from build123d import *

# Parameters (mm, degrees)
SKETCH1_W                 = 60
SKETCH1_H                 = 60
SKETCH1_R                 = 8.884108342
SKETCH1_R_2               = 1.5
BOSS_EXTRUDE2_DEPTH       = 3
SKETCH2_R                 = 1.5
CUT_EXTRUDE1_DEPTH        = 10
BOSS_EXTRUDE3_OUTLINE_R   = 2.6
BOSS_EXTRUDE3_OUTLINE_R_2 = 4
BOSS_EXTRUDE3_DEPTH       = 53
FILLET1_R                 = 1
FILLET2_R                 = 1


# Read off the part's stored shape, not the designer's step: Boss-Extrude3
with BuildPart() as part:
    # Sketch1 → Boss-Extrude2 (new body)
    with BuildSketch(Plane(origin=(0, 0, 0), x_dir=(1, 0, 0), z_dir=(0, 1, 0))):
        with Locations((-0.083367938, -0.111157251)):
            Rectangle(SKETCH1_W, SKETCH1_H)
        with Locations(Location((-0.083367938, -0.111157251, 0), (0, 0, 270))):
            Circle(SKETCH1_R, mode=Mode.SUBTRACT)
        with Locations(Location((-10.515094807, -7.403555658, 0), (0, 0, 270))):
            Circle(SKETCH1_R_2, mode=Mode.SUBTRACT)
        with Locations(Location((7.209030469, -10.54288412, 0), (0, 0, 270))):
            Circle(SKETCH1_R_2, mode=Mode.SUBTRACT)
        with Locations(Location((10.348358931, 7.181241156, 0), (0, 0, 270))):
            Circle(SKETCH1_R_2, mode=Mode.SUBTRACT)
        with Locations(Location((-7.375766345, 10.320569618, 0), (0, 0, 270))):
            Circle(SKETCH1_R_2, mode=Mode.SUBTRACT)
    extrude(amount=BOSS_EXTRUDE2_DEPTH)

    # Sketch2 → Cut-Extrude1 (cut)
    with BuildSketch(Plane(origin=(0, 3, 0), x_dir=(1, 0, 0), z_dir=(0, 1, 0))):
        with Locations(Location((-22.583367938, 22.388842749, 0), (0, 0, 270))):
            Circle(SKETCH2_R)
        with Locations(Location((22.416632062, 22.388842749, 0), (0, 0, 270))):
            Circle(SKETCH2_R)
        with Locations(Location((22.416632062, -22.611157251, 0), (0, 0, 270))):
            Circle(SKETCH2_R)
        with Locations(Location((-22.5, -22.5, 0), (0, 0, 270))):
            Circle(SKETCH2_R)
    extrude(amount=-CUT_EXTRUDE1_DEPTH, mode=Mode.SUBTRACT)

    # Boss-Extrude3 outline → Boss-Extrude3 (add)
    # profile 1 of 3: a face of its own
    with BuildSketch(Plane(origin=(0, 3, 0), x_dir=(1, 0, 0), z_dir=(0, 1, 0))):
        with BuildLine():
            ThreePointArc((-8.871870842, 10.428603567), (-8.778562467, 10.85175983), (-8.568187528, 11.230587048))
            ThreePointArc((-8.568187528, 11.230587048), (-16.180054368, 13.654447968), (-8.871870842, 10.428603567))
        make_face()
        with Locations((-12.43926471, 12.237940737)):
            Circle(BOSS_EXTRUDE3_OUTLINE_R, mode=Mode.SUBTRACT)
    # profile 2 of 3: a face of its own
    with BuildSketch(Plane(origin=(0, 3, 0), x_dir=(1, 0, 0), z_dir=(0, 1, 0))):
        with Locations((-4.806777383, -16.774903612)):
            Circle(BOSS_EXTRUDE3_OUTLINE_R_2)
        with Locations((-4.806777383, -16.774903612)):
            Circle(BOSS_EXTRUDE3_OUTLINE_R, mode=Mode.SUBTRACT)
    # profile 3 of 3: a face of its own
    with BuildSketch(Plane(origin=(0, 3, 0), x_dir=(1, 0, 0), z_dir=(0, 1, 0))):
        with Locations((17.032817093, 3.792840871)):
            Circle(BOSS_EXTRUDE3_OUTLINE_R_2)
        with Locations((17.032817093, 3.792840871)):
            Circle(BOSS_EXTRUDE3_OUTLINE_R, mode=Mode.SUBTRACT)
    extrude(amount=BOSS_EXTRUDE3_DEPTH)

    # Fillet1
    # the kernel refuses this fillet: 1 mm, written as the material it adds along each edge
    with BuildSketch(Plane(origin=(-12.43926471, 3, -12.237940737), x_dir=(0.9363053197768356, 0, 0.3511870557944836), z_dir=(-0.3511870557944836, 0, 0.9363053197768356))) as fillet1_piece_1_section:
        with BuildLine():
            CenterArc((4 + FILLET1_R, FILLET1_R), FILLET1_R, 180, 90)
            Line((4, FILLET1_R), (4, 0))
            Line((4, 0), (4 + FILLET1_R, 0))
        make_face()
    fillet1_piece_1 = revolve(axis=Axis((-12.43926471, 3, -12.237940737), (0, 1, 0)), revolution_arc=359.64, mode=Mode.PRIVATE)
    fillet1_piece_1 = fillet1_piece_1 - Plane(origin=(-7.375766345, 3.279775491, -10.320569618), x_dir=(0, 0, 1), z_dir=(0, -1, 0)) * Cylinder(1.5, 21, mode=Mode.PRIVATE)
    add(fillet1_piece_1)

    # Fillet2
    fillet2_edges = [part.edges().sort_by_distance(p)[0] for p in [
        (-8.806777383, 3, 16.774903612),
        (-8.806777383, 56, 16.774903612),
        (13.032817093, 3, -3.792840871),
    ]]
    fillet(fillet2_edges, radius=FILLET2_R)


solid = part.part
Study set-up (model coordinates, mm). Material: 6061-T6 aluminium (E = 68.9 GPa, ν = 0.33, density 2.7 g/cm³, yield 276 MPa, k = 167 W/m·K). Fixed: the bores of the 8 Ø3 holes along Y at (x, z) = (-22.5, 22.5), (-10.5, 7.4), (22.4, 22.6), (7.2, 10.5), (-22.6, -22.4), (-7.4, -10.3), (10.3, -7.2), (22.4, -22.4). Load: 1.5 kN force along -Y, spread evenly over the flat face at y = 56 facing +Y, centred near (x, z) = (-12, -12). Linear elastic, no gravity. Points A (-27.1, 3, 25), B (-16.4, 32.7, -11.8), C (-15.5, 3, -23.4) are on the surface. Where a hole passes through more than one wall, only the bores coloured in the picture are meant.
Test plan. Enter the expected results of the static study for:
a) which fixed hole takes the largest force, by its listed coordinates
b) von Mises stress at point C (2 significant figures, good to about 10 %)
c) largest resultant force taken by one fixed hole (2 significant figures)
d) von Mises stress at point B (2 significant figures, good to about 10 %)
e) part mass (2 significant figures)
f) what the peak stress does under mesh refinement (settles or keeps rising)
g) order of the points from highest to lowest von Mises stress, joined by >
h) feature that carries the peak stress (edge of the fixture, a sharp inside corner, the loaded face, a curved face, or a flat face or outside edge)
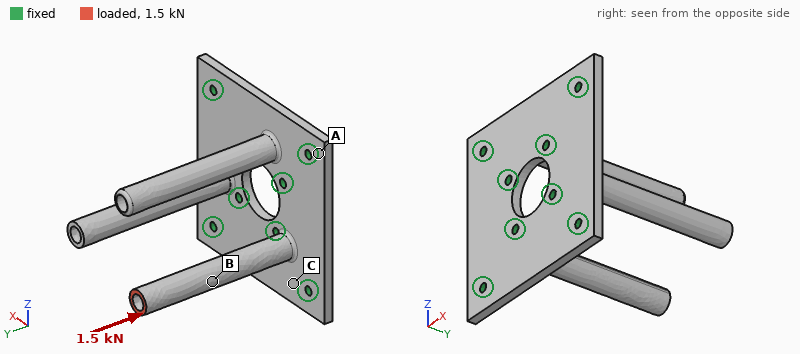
(-7.4, -10.3)
15 MPa
1.1 kN
52 MPa
39 g
keeps rising
B > C > A
edge of the fixture
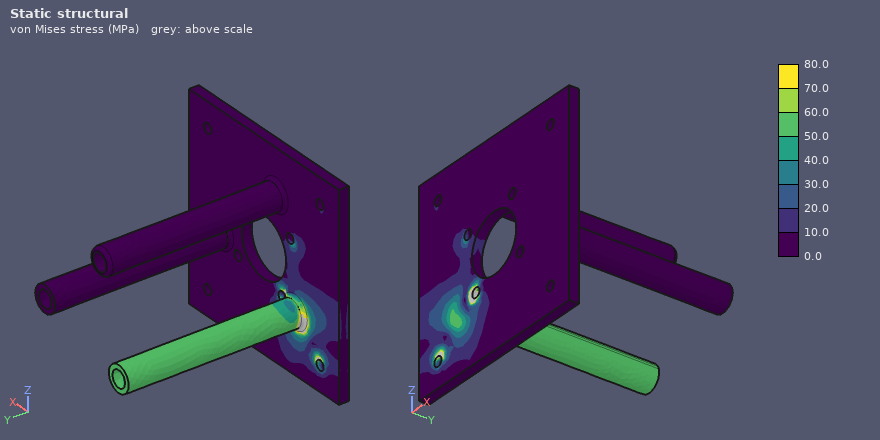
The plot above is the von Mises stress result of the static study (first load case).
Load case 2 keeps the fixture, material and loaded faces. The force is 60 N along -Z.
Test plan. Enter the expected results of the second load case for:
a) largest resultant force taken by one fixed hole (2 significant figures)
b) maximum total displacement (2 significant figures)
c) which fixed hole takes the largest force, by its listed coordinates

99 N
0.34 mm
(-22.6, -22.4)
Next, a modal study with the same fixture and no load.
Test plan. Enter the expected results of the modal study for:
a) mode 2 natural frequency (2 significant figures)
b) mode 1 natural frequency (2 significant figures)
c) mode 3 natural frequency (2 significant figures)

1800 Hz
1800 Hz
2000 Hz
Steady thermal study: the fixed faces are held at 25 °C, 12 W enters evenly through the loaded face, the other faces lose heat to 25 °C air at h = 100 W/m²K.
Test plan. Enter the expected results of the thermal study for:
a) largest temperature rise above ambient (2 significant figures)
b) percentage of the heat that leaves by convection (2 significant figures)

78 K
63 %
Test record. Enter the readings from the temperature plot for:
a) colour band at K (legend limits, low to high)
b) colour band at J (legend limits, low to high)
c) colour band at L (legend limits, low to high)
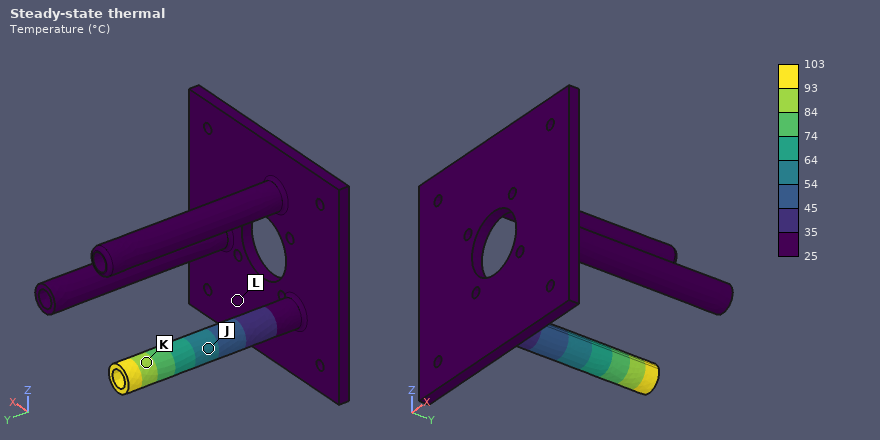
84 to 93 °C
54 to 64 °C
25 to 35 °C
